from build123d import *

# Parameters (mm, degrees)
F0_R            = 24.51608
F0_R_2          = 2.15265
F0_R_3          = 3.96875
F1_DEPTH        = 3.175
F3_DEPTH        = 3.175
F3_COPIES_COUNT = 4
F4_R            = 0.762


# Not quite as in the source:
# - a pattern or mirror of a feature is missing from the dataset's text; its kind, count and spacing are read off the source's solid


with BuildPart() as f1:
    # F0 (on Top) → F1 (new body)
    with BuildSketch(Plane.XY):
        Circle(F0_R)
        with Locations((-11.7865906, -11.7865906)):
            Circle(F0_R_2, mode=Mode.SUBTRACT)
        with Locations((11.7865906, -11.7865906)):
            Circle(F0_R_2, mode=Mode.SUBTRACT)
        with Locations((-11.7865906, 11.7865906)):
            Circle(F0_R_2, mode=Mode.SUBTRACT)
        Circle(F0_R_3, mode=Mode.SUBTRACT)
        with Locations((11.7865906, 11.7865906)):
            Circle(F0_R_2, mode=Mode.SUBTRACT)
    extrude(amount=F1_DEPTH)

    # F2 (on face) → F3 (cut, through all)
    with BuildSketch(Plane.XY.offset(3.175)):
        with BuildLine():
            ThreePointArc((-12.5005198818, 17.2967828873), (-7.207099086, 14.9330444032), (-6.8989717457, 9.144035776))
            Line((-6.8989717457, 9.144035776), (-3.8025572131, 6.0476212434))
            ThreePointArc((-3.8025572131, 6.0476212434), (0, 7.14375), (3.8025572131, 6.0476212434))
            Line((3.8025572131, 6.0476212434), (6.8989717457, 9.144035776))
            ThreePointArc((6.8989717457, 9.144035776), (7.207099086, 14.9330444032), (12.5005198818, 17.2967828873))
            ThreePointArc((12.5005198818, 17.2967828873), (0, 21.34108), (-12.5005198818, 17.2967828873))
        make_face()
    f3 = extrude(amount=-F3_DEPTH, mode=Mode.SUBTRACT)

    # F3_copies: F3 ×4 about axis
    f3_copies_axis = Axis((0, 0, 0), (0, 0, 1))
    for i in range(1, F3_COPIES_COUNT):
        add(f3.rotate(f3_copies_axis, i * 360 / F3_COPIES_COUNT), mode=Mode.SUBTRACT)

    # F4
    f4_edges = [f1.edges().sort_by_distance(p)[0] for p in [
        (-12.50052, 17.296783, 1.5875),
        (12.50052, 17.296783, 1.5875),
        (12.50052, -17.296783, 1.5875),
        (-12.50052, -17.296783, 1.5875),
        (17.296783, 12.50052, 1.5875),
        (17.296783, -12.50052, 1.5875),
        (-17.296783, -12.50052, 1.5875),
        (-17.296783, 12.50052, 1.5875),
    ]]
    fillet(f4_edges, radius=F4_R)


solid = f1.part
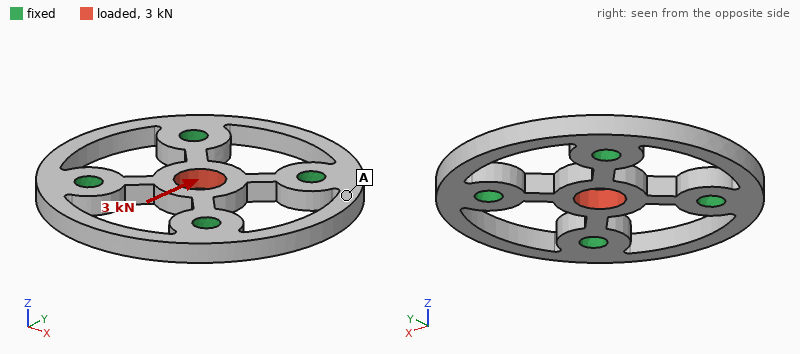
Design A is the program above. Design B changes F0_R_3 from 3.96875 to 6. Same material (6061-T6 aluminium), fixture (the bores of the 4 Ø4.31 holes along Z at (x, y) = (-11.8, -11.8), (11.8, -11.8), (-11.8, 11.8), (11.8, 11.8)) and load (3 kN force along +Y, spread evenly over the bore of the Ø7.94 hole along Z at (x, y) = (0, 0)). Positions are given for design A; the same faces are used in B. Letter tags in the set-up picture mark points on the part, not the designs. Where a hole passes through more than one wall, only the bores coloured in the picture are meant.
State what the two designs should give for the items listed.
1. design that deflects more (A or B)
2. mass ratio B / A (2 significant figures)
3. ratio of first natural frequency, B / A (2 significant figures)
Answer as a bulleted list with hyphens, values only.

- B
- 0.93
- 1.00
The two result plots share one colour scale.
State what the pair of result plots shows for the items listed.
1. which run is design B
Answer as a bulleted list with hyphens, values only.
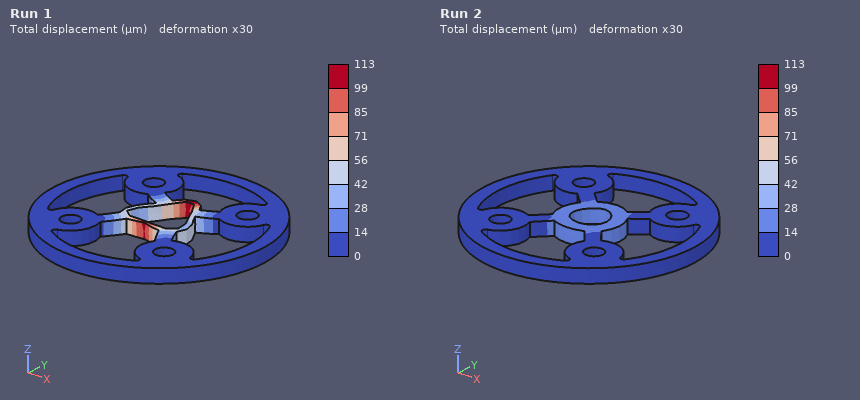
- Run 1
